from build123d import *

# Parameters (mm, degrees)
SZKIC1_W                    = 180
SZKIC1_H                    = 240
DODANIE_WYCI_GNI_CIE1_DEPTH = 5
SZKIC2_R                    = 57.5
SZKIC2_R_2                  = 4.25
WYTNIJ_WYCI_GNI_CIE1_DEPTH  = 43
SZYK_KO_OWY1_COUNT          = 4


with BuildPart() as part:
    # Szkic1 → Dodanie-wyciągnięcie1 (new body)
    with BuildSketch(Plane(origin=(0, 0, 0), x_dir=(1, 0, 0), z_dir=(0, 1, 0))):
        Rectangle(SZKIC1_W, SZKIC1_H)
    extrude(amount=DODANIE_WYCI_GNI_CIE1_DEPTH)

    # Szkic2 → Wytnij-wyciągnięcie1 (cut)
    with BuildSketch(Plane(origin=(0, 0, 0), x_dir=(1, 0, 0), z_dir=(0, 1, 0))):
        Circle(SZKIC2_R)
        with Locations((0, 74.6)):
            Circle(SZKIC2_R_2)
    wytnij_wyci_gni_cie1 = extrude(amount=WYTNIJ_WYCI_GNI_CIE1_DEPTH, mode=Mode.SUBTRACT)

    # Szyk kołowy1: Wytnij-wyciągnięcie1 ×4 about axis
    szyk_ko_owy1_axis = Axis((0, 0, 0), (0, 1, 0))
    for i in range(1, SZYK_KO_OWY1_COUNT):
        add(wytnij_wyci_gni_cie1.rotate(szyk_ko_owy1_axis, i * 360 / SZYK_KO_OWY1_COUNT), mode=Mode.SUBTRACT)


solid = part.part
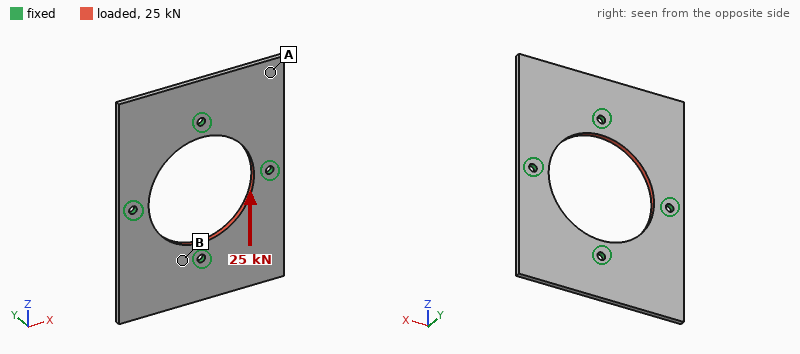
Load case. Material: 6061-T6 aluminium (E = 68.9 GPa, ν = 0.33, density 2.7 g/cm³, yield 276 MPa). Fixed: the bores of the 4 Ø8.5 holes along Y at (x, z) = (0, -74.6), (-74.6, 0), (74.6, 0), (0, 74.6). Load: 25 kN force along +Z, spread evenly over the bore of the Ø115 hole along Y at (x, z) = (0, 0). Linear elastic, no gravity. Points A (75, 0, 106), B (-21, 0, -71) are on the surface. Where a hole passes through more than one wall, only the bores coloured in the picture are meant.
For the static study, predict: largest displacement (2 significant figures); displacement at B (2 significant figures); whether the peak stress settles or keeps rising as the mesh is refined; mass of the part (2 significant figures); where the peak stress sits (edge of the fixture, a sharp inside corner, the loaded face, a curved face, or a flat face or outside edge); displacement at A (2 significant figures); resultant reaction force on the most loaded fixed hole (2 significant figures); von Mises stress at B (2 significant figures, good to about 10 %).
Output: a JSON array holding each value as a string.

["21 µm", "11 µm", "keeps rising", "440 g", "edge of the fixture", "15 µm", "7.0 kN", "15 MPa"]
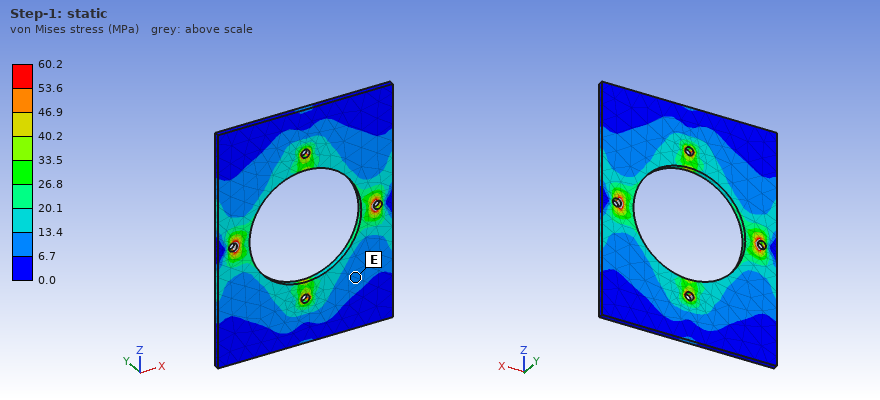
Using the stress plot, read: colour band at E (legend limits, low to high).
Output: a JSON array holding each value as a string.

["6.7 to 13.4 MPa"]
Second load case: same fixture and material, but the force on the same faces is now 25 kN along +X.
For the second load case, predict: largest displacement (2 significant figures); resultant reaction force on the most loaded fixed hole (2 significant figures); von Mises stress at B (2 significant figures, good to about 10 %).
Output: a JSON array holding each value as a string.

["23 µm", "7.3 kN", "21 MPa"]
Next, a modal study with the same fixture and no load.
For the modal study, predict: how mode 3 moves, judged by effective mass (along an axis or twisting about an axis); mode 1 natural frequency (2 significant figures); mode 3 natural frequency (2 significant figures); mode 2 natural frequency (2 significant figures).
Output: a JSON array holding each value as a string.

["along Y", "620 Hz", "700 Hz", "620 Hz"]
